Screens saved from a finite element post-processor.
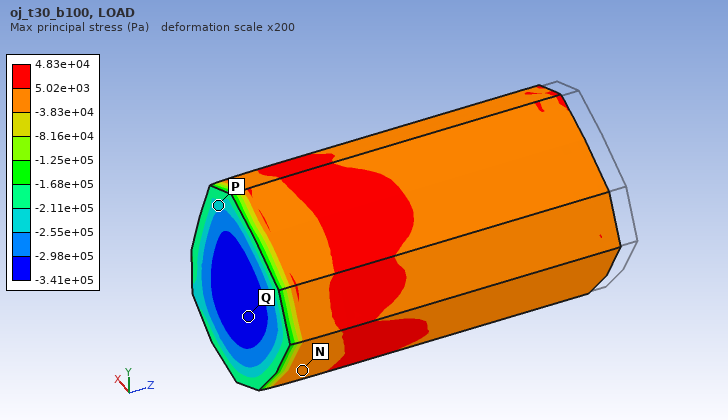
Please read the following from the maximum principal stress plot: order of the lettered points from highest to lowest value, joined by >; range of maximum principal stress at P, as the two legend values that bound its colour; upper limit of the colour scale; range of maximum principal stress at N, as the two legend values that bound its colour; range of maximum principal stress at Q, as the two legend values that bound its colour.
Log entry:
N > P > Q
-2.55e+05 to -2.11e+05 Pa
4.83e+04 Pa
-3.83e+04 to 5.02e+03 Pa
-3.41e+05 to -2.98e+05 Pa
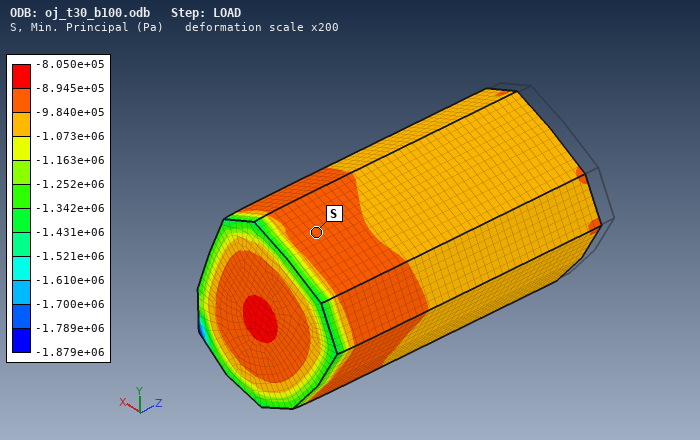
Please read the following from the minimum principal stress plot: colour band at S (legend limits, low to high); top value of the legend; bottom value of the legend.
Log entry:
-9.840e+05 to -8.945e+05 Pa
-8.050e+05 Pa
-1.879e+06 Pa
